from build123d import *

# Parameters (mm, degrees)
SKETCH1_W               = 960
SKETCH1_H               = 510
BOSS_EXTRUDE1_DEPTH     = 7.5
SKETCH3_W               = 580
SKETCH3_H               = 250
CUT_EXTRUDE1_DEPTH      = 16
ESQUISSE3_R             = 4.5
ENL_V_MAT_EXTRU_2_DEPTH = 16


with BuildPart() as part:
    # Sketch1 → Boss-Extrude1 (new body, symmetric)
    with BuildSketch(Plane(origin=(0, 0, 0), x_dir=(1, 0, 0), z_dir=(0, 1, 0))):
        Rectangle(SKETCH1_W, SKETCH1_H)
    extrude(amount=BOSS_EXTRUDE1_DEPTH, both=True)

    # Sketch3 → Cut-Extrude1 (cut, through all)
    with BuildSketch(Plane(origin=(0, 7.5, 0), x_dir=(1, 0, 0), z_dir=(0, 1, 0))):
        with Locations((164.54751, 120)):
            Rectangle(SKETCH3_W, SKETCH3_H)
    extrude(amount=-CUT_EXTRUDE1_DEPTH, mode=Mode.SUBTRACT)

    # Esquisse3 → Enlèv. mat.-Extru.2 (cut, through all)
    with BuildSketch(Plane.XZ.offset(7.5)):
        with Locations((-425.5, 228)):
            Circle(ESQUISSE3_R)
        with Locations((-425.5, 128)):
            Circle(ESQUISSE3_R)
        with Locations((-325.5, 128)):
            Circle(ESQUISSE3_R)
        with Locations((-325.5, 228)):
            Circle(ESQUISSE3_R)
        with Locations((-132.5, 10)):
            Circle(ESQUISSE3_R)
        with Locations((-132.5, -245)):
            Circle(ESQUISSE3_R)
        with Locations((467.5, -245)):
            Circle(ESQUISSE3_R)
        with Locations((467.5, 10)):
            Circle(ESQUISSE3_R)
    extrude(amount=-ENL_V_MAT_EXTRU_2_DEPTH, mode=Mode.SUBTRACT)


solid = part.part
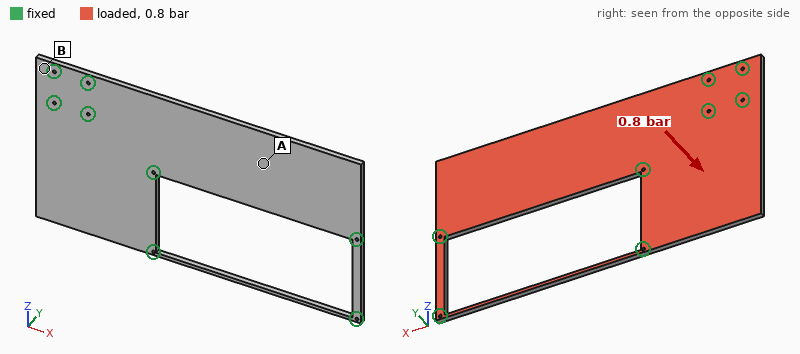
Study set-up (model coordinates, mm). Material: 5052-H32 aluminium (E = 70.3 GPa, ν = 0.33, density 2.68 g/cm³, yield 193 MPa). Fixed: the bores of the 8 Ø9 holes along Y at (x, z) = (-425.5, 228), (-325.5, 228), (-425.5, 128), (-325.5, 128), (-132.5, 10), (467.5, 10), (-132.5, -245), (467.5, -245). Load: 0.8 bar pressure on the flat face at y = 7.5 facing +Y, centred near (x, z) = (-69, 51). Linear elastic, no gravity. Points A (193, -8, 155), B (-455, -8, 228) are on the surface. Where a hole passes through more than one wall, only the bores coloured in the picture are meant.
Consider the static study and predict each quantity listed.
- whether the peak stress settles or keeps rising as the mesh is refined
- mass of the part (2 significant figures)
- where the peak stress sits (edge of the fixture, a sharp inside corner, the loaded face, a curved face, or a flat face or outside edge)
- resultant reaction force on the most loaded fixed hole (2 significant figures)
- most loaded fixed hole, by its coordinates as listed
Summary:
keeps rising
14 kg
edge of the fixture
9.0 kN
(-132.5, 10)
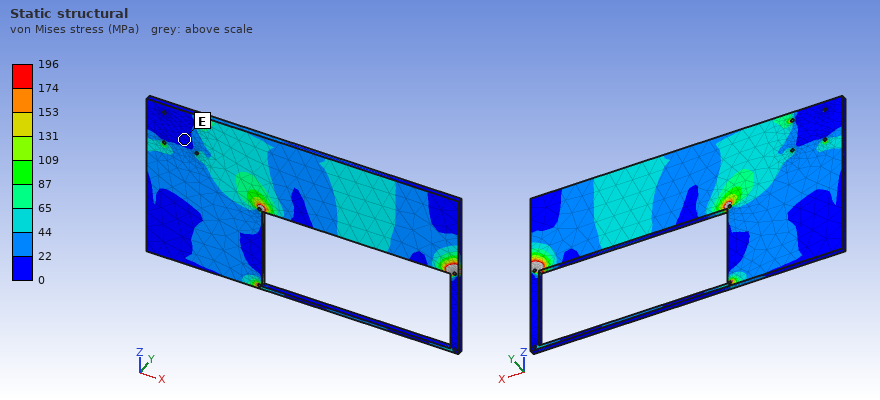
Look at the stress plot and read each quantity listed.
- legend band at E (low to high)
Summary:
0 to 22 MPa
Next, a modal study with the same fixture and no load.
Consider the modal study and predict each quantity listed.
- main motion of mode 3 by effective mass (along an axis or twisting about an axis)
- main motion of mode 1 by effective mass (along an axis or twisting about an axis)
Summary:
along Y
along Y
